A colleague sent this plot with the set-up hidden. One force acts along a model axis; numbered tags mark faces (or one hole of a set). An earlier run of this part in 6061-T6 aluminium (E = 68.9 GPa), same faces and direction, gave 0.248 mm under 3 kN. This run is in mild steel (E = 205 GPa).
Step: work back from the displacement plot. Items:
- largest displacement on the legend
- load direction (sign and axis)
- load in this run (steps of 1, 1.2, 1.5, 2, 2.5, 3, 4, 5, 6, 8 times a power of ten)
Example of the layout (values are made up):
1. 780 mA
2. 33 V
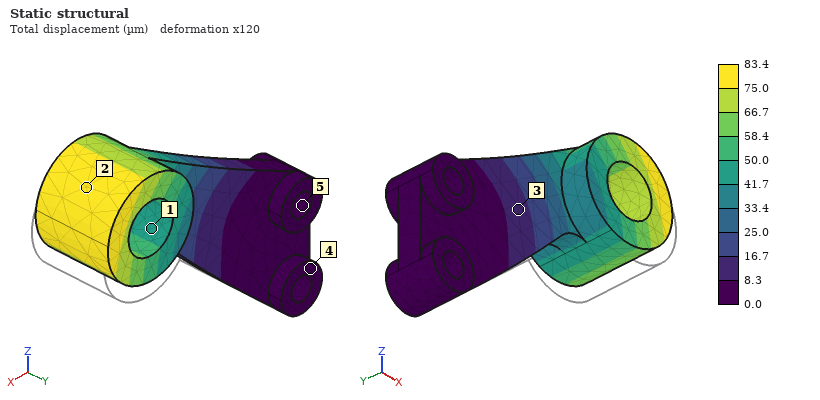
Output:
1. 83.4 µm
2. +Z
3. 3 kN
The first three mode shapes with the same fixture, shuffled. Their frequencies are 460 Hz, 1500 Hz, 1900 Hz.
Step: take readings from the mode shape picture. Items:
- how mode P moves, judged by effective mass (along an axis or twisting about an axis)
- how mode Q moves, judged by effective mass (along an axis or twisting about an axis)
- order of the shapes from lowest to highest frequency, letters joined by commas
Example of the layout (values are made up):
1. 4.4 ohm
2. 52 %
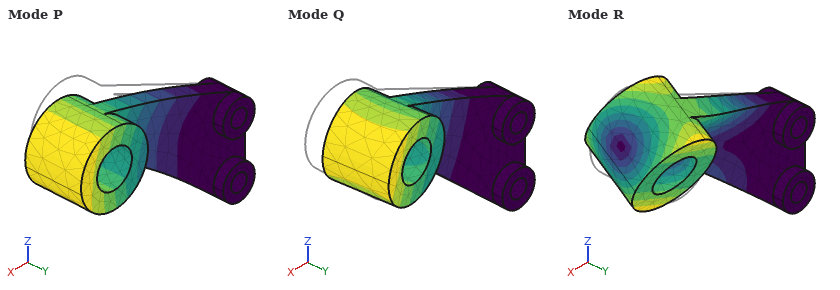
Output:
1. along Z
2. along Y
3. Q, P, R
